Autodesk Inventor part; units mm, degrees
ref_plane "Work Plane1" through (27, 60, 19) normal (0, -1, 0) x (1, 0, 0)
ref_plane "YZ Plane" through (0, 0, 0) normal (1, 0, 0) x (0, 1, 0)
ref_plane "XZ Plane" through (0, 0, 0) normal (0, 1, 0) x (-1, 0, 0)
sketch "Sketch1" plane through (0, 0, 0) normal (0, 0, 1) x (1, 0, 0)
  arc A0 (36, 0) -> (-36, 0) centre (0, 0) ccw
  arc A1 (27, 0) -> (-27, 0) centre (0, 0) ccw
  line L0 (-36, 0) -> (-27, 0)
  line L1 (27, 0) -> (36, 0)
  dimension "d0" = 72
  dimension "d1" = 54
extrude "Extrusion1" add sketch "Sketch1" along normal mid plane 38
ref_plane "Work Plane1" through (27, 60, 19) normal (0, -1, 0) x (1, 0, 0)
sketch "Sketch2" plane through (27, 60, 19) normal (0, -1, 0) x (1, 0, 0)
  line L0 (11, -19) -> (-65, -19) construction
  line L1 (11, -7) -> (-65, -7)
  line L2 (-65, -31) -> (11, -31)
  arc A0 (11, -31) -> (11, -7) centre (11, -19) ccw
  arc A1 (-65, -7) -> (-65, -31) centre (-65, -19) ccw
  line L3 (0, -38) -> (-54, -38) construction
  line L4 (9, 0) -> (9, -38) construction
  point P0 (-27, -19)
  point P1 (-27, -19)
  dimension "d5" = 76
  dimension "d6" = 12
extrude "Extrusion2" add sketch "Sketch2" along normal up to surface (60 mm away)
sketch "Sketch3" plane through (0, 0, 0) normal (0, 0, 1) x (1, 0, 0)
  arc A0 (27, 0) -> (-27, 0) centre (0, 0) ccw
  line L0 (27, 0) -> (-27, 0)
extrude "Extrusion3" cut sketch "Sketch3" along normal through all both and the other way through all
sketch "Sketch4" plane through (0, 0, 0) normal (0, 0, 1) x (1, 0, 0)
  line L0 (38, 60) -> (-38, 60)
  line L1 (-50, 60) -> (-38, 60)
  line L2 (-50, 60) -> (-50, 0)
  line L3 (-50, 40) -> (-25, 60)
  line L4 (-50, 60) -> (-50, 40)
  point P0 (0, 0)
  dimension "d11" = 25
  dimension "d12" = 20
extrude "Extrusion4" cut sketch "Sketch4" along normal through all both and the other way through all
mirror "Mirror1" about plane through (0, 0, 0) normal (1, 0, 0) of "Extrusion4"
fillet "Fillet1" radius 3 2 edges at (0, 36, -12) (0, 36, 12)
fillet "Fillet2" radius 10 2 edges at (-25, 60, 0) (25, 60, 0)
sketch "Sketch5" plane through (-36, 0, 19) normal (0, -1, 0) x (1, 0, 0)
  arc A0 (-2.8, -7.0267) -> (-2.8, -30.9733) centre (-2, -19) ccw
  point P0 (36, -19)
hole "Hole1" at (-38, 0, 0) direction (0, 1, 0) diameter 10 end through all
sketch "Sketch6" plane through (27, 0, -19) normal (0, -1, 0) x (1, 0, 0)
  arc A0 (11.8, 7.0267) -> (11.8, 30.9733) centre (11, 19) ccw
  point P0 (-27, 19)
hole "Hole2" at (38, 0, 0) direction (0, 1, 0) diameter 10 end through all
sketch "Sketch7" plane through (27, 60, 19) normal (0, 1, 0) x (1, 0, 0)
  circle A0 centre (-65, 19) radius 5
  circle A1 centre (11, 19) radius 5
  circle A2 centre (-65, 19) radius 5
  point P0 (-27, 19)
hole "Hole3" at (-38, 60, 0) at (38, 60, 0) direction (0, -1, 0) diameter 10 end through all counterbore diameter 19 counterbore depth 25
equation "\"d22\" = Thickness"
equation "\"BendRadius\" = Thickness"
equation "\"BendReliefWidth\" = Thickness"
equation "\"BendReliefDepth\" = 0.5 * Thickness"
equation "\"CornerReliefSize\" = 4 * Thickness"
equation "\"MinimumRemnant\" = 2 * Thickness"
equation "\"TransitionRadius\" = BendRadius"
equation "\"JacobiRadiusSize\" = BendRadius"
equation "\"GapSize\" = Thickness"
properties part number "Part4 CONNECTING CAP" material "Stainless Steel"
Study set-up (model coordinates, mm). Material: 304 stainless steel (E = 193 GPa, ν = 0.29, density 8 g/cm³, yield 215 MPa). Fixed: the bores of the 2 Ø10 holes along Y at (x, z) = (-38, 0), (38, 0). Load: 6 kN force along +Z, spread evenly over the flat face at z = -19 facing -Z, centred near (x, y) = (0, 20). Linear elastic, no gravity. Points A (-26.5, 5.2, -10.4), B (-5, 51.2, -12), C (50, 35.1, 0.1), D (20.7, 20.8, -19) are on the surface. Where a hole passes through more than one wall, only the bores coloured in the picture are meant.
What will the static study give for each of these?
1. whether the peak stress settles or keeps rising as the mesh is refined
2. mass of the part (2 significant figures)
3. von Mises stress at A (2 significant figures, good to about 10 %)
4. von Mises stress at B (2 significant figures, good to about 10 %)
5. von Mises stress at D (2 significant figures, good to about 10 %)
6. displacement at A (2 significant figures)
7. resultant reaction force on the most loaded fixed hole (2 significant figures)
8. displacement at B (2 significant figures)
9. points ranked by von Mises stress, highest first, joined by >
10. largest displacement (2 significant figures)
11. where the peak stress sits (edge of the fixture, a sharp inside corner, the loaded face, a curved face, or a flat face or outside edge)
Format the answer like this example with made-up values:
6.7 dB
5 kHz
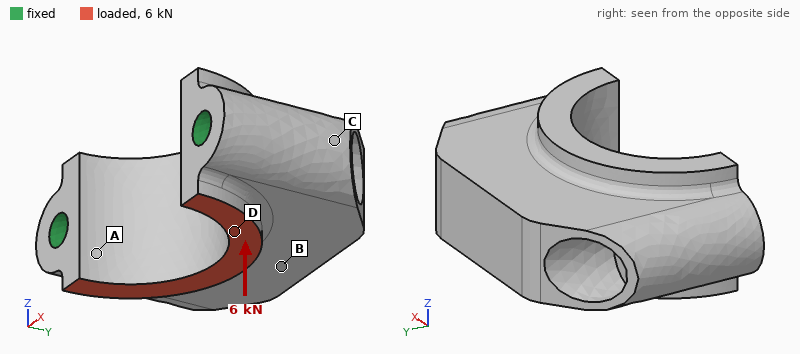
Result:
keeps rising
790 g
8.2 MPa
2.8 MPa
5.9 MPa
0.84 µm
3.0 kN
1.9 µm
A > D > B > C
2.2 µm
edge of the fixture
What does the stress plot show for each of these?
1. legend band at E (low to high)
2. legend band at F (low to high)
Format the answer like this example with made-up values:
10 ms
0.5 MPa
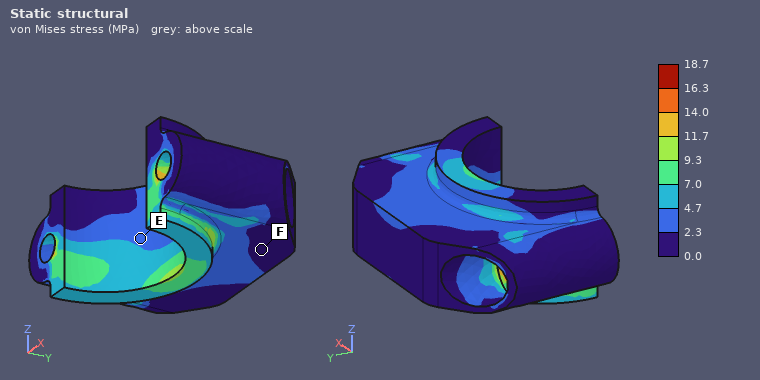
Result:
2.3 to 4.7 MPa
0.0 to 2.3 MPa
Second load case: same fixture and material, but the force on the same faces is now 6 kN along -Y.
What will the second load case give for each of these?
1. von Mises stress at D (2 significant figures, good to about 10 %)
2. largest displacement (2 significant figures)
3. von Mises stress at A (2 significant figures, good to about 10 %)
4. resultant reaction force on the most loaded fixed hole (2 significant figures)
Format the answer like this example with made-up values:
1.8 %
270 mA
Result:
20 MPa
5.5 µm
13 MPa
3.2 kN
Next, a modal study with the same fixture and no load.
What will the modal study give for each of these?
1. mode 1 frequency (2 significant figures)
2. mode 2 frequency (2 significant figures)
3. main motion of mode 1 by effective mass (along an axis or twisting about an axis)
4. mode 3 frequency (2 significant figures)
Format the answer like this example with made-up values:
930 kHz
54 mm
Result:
7700 Hz
16 kHz
along Z
16 kHz
